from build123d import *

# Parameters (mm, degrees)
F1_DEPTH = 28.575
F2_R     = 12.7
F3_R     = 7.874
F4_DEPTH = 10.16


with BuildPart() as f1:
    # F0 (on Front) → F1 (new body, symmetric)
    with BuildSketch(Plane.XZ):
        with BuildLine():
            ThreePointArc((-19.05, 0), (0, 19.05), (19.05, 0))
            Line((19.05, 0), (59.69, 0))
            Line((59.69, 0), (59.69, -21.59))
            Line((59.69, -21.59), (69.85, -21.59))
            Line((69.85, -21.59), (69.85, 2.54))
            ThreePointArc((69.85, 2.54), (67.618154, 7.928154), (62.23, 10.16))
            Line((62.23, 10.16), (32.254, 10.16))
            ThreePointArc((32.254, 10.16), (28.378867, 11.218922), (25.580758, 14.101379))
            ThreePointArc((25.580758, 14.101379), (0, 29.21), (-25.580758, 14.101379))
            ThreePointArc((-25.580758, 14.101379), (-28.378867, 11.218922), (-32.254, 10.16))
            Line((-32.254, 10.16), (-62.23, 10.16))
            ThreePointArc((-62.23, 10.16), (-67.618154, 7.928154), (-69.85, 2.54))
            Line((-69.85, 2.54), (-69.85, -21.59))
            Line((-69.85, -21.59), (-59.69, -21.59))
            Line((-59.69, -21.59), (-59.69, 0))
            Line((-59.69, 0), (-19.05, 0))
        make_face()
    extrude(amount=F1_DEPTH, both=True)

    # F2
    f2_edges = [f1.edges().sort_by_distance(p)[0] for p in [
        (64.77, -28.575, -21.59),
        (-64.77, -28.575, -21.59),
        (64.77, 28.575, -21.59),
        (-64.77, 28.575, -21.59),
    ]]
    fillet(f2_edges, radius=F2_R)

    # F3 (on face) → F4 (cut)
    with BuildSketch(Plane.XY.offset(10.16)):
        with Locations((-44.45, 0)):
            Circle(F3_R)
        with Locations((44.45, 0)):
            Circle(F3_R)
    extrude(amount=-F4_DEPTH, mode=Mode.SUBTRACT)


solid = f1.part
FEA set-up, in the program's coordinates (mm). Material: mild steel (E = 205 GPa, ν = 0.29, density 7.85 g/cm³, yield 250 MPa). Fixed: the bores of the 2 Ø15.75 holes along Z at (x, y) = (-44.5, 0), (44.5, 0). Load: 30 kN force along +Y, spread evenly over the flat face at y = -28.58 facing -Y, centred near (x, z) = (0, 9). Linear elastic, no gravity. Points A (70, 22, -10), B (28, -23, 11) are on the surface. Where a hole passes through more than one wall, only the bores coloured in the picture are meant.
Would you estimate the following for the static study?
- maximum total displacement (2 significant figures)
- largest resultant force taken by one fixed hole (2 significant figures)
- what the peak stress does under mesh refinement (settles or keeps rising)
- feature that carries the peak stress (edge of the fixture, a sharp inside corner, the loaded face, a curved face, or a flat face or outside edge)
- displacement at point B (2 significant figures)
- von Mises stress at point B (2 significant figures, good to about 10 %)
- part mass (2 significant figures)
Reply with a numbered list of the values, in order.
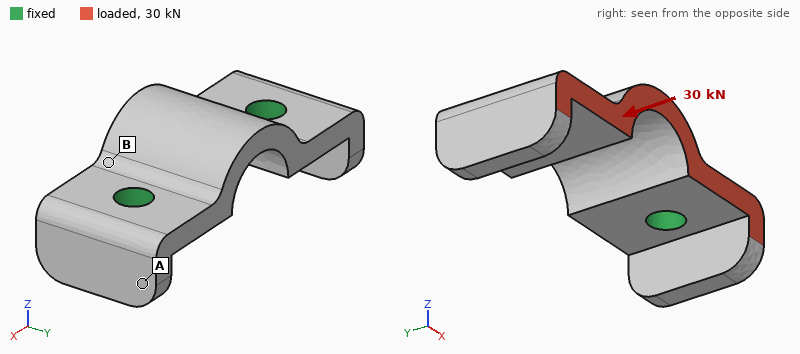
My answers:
1. 33 µm
2. 15 kN
3. keeps rising
4. edge of the fixture
5. 15 µm
6. 51 MPa
7. 870 g
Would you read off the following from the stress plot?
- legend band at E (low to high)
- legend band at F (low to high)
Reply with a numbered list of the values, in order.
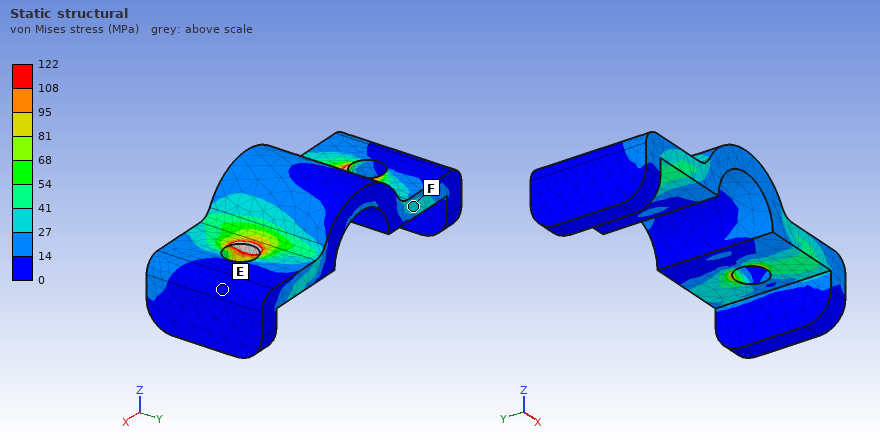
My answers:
1. 0 to 14 MPa
2. 27 to 41 MPa
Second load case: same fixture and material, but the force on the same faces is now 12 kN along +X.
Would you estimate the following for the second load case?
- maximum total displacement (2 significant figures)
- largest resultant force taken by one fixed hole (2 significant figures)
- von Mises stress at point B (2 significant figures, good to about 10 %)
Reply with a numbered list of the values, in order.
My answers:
1. 10 µm
2. 6.4 kN
3. 31 MPa
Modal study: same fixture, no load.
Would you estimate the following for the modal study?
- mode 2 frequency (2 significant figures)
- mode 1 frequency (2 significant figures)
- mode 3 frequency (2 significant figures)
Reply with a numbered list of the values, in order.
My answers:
1. 5900 Hz
2. 5400 Hz
3. 5900 Hz
